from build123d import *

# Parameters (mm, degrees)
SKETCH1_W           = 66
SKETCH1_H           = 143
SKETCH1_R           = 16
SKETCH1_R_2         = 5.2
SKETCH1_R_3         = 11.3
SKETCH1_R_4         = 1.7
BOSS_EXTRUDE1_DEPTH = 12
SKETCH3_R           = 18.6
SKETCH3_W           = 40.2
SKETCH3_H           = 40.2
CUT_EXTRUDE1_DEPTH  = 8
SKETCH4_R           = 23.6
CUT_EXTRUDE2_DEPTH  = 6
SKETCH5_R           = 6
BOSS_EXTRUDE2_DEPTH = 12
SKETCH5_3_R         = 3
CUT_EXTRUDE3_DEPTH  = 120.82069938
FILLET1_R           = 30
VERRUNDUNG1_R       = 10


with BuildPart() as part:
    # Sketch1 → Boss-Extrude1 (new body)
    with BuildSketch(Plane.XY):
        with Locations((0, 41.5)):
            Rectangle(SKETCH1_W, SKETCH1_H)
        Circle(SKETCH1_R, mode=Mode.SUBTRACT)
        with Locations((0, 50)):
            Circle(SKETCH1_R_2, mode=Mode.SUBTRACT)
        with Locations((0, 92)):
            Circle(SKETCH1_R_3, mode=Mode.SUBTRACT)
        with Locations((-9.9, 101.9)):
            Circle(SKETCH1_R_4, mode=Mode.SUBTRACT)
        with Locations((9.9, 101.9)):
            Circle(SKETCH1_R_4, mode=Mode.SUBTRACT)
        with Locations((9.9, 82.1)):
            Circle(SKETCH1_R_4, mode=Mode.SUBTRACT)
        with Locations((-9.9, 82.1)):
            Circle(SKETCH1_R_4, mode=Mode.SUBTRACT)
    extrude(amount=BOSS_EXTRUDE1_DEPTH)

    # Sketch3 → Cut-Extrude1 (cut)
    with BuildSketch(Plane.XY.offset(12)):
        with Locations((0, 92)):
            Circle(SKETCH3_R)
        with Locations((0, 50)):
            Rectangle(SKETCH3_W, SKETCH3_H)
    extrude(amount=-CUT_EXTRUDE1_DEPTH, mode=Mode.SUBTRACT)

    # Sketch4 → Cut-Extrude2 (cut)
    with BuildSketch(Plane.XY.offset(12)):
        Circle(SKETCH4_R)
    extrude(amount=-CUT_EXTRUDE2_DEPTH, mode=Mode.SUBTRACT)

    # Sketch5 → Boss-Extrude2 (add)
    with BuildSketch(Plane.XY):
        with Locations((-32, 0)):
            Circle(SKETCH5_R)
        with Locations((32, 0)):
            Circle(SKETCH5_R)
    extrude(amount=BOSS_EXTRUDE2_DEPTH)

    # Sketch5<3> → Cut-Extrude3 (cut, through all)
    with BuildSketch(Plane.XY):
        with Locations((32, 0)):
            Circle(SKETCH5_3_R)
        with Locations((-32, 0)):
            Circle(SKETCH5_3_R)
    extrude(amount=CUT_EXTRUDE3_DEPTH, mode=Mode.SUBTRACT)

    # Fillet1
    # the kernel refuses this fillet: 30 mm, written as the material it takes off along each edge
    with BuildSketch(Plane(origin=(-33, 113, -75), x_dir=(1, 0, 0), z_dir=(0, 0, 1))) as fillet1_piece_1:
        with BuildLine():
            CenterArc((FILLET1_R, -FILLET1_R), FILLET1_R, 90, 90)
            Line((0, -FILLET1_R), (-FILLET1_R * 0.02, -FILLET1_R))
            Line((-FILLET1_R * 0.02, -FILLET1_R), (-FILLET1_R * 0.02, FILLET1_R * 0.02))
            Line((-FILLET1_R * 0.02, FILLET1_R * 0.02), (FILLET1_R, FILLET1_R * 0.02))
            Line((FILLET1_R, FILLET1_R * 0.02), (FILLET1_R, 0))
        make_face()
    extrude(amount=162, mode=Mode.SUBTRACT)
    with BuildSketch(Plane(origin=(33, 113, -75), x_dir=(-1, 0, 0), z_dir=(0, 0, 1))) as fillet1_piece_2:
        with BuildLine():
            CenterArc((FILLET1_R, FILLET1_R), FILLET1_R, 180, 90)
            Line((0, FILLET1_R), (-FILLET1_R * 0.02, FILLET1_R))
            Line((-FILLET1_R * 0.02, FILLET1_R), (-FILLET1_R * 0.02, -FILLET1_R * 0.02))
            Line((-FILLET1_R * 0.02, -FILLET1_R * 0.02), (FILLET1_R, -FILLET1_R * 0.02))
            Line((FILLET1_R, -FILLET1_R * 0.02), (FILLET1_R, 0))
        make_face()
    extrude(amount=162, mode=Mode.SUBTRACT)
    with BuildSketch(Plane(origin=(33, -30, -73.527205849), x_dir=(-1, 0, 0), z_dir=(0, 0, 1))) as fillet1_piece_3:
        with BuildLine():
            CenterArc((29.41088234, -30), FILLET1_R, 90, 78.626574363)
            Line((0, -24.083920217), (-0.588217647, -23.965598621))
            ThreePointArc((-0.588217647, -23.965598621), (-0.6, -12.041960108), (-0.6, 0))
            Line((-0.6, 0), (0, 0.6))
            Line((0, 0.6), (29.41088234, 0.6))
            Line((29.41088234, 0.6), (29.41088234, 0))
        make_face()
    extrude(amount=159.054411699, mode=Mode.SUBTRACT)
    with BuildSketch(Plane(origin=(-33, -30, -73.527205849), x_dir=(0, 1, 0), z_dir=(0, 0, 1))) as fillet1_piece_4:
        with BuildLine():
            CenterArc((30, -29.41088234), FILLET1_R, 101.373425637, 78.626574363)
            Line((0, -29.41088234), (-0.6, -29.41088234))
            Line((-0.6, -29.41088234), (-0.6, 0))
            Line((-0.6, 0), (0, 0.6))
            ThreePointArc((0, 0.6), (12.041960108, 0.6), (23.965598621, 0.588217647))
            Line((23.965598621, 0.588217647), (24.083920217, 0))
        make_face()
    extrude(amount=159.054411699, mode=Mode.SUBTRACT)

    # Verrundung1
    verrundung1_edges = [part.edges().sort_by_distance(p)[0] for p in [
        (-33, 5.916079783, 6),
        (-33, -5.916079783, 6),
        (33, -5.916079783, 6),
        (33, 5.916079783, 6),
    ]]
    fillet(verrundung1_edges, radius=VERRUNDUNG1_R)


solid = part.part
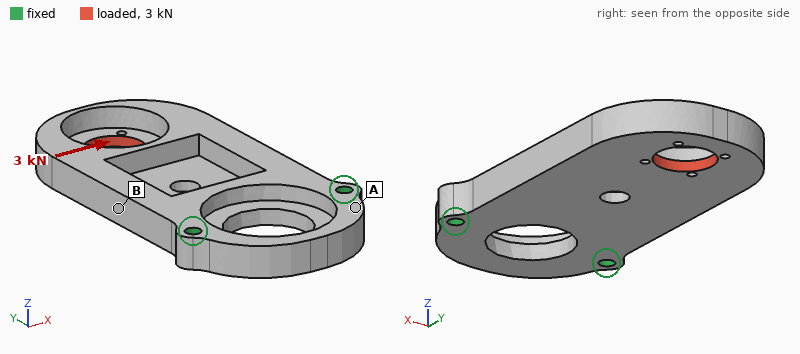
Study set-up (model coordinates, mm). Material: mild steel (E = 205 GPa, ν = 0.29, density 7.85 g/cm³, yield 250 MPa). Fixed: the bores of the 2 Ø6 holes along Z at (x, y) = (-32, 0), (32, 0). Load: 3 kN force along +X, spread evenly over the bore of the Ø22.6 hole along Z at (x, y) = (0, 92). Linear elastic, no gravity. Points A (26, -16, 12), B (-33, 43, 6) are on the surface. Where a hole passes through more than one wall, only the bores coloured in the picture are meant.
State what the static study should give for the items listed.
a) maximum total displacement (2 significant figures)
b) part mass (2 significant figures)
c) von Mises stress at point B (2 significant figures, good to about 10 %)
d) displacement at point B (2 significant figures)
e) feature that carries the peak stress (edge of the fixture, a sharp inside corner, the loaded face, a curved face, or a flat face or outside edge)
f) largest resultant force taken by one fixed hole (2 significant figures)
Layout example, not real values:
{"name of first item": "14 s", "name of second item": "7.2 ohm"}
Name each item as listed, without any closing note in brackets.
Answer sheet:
{"maximum total displacement": "41 µm", "part mass": "520 g", "von Mises stress at point B": "23 MPa", "displacement at point B": "12 µm", "feature that carries the peak stress": "a curved face", "largest resultant force taken by one fixed hole": "4.6 kN"}
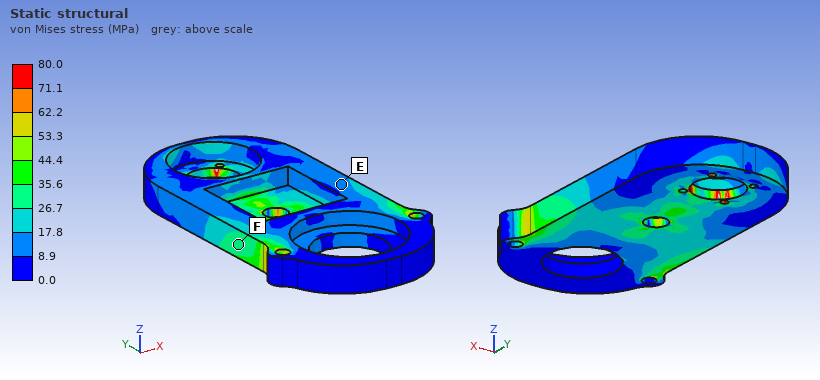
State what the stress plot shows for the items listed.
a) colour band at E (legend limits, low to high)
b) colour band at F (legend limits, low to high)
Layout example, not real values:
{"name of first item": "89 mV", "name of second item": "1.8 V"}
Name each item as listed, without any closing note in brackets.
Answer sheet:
{"colour band at E": "8.9 to 17.8 MPa", "colour band at F": "26.7 to 35.6 MPa"}
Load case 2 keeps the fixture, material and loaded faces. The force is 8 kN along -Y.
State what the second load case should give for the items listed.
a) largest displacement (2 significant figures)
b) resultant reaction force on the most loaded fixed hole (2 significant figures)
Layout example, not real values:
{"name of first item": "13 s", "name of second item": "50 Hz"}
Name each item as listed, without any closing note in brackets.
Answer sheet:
{"largest displacement": "0.15 mm", "resultant reaction force on the most loaded fixed hole": "4.1 kN"}
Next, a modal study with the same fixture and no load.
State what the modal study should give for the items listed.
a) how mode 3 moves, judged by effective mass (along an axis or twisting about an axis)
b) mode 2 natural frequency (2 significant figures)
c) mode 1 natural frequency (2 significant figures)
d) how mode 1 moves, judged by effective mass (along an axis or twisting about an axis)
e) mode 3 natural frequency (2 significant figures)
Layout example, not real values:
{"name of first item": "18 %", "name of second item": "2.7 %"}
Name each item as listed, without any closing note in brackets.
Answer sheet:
{"how mode 3 moves, judged by effective mass": "along X", "mode 2 natural frequency": "2000 Hz", "mode 1 natural frequency": "760 Hz", "how mode 1 moves, judged by effective mass": "along Z", "mode 3 natural frequency": "4000 Hz"}
